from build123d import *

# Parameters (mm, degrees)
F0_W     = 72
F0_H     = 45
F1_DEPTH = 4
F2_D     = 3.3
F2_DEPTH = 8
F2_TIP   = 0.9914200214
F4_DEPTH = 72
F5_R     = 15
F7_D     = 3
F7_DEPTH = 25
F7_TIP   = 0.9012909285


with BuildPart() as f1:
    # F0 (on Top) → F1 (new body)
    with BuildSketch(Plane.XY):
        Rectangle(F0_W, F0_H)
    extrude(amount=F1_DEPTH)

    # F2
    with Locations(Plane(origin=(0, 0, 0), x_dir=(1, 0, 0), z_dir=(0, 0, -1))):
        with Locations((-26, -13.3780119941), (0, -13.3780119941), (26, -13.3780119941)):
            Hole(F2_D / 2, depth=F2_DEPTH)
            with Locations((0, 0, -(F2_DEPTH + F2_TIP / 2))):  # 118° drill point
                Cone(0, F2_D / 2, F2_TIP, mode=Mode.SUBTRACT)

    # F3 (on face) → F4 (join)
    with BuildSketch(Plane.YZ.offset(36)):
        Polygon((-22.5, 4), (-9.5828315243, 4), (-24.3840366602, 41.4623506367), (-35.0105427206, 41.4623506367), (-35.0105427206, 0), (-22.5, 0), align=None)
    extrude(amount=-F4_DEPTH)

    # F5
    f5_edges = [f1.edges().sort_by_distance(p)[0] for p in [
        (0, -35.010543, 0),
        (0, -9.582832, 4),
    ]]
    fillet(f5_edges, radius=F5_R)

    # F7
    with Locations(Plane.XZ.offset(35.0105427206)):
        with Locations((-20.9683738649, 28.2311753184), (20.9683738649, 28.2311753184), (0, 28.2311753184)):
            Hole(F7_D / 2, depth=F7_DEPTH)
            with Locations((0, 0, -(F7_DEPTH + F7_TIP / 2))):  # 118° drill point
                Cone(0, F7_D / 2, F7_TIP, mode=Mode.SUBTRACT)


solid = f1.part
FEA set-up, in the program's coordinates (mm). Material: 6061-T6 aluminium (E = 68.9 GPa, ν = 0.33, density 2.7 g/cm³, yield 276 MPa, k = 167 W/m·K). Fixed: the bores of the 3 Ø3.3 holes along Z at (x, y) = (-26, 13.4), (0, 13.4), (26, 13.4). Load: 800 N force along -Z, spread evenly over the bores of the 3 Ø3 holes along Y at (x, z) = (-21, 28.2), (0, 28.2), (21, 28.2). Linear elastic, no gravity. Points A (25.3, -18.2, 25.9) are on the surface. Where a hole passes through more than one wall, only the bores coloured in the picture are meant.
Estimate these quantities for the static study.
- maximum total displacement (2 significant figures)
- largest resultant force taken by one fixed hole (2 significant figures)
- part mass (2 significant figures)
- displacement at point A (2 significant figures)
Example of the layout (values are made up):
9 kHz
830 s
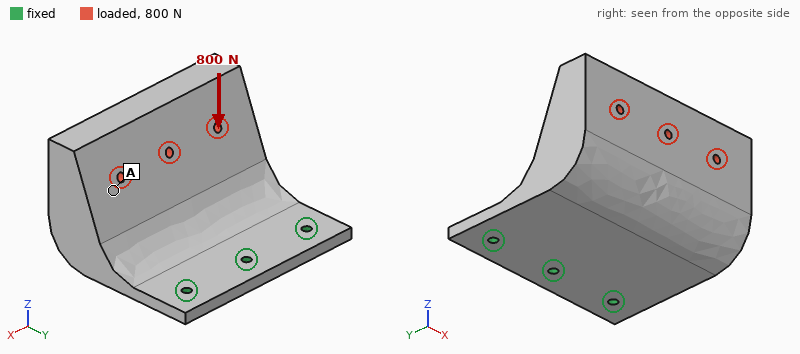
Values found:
1.0 mm
280 N
170 g
0.62 mm
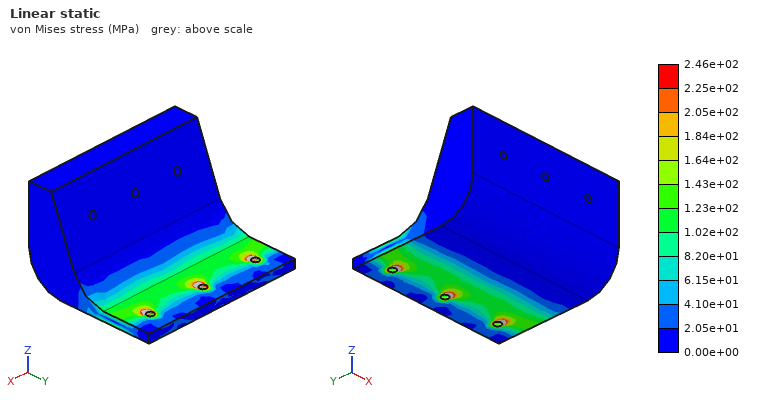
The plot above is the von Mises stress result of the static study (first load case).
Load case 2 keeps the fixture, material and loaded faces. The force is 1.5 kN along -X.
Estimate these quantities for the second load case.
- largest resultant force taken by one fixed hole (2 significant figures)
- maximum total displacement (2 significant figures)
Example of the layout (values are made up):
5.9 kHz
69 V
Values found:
1.4 kN
0.17 mm
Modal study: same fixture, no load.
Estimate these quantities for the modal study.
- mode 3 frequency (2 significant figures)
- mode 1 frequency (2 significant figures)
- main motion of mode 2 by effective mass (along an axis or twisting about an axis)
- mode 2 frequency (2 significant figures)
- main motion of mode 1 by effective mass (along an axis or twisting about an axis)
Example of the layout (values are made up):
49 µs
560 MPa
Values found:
3600 Hz
430 Hz
along X
1600 Hz
along Z
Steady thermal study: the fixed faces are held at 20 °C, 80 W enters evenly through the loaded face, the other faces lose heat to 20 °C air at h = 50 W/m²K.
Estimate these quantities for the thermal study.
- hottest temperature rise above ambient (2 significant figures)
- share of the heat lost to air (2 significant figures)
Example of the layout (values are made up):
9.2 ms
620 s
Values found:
45 K
27 %
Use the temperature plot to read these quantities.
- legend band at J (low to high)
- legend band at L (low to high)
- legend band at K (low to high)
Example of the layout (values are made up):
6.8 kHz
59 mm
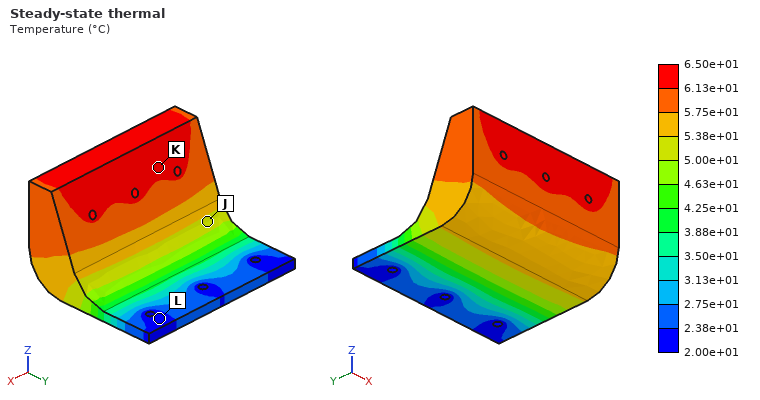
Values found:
5.00e+01 to 5.38e+01 °C
2.00e+01 to 2.38e+01 °C
6.13e+01 to 6.50e+01 °C
